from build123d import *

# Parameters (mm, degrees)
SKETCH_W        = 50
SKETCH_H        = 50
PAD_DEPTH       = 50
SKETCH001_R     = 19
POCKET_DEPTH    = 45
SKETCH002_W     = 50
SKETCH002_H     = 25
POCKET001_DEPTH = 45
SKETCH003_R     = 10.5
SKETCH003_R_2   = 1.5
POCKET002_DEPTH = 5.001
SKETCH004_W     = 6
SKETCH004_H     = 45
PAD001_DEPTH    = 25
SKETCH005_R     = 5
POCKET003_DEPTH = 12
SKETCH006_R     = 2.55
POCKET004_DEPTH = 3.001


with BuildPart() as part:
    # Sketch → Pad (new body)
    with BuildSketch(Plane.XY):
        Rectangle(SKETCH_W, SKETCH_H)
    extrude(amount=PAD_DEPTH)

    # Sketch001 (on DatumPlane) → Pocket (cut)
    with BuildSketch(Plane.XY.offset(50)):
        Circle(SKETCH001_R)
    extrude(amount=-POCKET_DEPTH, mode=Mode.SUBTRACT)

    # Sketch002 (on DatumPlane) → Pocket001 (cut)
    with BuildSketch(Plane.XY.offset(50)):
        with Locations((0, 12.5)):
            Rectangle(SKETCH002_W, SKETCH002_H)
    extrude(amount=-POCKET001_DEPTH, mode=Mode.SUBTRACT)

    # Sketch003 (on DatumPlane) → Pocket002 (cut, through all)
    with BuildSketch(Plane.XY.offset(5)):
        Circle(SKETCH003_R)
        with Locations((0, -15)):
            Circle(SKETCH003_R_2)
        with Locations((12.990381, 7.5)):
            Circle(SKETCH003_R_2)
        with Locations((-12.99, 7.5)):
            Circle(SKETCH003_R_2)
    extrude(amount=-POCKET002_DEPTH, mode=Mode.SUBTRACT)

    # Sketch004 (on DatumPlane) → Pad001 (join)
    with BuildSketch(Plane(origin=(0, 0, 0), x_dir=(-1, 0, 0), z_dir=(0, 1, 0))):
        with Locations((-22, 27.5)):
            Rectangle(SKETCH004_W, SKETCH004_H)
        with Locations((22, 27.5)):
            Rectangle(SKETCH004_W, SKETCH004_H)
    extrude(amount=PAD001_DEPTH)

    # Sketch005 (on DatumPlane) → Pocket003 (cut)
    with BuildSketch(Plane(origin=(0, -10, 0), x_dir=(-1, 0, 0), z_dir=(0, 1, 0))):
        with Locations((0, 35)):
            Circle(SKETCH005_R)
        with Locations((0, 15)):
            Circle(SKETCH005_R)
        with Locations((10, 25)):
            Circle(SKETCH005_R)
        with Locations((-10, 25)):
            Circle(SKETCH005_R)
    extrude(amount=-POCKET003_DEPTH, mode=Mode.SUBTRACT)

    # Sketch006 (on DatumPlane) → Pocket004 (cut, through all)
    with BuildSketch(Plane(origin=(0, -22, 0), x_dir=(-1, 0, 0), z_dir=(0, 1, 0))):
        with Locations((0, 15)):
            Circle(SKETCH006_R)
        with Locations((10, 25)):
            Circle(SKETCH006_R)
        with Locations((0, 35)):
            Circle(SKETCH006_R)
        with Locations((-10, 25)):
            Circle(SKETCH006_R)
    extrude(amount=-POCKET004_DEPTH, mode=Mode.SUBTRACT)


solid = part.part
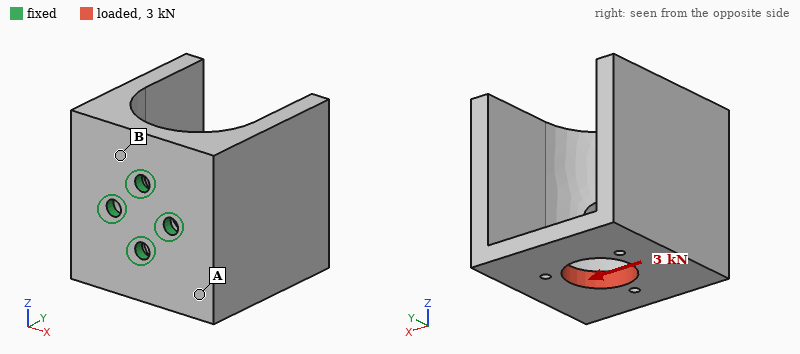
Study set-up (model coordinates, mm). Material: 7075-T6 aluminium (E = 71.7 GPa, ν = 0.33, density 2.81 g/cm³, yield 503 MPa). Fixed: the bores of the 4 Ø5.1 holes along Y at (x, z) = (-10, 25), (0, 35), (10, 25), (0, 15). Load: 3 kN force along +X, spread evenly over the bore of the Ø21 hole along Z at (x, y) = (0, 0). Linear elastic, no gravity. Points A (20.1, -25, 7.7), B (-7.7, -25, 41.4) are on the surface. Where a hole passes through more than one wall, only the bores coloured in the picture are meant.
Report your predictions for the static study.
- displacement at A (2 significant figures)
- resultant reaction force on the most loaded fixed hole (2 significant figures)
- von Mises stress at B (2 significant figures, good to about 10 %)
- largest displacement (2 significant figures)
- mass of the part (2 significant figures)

0.050 mm
3.2 kN
35 MPa
0.18 mm
150 g
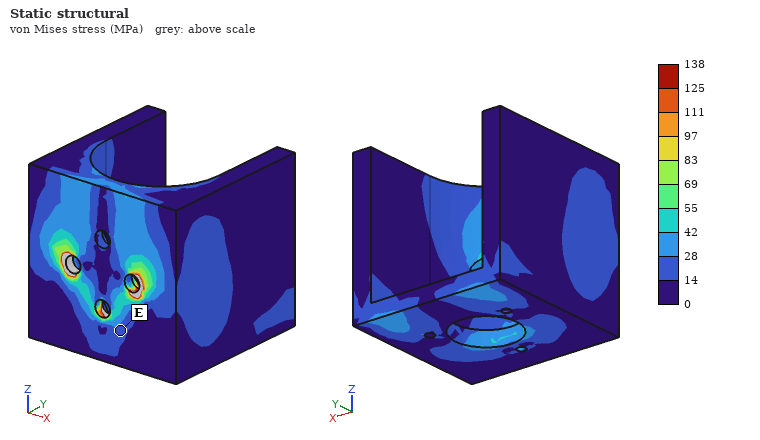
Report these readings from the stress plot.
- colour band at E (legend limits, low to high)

14 to 28 MPa
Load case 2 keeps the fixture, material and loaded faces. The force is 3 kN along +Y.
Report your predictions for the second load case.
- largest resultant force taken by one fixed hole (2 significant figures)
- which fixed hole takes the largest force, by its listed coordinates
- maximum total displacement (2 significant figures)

3.3 kN
(0, 15)
0.10 mm
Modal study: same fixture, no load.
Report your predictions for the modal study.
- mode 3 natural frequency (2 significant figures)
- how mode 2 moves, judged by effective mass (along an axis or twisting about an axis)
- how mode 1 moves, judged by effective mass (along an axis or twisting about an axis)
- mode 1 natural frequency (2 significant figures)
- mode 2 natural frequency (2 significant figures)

4100 Hz
along Z
along X
2400 Hz
2600 Hz
